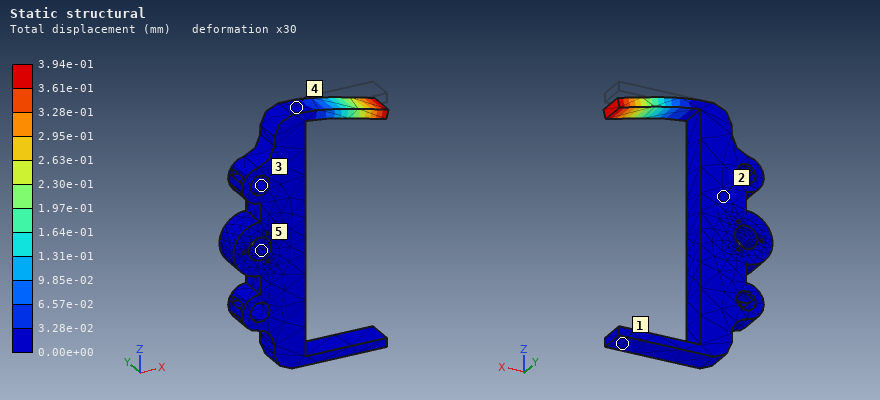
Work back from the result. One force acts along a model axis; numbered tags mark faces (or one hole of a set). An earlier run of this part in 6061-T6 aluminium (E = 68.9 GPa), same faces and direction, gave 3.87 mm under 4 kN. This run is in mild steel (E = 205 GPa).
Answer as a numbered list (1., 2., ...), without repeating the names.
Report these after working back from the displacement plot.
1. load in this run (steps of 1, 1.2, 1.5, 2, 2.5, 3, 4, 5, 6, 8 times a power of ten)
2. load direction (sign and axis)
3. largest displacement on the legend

1. 1.2 kN
2. -Z
3. 3.94e-01 mm
